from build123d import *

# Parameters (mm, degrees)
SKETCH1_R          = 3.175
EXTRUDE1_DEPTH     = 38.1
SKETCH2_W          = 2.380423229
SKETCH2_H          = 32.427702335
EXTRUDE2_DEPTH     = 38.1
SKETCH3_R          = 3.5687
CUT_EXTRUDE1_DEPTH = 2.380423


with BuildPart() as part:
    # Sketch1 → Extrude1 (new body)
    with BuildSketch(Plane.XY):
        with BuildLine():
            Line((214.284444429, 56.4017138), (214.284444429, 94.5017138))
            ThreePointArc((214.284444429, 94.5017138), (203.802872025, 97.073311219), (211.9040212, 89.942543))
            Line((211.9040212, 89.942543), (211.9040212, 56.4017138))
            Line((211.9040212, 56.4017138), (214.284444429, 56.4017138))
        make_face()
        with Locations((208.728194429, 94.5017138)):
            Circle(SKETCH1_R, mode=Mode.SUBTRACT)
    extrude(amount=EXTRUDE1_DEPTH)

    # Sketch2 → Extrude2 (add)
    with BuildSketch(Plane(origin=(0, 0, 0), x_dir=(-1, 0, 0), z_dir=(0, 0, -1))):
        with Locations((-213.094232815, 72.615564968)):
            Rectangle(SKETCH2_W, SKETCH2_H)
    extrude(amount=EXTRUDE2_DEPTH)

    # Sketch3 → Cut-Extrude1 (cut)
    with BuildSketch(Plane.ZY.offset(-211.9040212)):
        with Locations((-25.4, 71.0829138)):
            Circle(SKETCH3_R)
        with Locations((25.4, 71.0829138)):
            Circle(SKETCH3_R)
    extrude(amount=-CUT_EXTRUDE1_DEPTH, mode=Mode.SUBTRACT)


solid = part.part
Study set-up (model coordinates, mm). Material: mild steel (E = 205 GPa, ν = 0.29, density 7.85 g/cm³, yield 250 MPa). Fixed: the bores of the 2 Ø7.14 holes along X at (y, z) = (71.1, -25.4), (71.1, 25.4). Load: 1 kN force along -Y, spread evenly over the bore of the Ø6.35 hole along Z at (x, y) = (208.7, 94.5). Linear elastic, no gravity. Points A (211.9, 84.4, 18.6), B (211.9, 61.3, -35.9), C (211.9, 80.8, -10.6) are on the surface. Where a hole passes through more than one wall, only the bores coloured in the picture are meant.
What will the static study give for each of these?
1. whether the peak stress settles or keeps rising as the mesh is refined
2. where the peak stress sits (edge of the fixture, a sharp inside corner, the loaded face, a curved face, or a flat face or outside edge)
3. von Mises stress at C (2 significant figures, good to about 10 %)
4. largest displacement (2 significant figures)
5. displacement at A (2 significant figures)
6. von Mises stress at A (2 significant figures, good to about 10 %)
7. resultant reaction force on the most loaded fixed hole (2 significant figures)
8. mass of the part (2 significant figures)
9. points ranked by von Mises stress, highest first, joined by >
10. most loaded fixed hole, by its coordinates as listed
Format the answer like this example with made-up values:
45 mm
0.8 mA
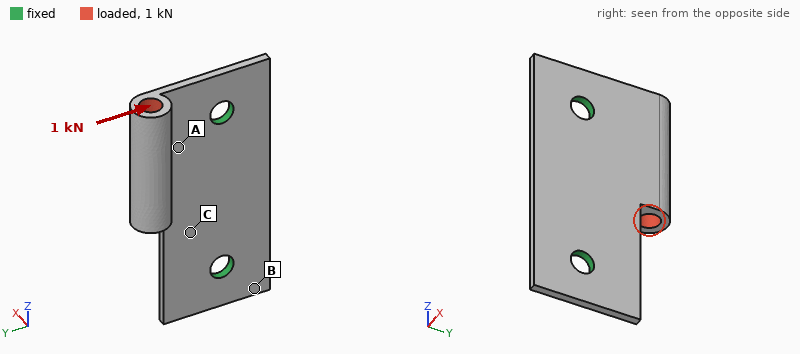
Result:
keeps rising
a sharp inside corner
46 MPa
0.15 mm
0.031 mm
110 MPa
870 N
66 g
A > C > B
(71.1, 25.4)
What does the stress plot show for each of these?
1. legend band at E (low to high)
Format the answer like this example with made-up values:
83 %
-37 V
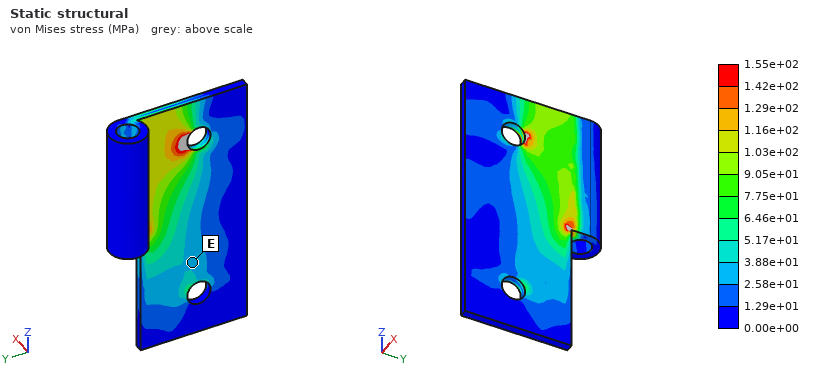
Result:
2.58e+01 to 3.88e+01 MPa
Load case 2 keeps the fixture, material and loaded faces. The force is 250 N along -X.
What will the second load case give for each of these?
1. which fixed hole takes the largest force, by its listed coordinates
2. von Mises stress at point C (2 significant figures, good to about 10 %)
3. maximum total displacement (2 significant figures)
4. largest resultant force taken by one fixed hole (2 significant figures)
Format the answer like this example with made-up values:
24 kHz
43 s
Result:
(71.1, 25.4)
41 MPa
0.13 mm
220 N
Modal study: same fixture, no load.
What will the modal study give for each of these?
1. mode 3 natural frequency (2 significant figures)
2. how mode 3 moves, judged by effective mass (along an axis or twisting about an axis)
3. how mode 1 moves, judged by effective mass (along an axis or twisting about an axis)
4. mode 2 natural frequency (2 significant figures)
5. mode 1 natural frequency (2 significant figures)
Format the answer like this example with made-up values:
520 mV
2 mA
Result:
5500 Hz
along X
along X
3600 Hz
1700 Hz
